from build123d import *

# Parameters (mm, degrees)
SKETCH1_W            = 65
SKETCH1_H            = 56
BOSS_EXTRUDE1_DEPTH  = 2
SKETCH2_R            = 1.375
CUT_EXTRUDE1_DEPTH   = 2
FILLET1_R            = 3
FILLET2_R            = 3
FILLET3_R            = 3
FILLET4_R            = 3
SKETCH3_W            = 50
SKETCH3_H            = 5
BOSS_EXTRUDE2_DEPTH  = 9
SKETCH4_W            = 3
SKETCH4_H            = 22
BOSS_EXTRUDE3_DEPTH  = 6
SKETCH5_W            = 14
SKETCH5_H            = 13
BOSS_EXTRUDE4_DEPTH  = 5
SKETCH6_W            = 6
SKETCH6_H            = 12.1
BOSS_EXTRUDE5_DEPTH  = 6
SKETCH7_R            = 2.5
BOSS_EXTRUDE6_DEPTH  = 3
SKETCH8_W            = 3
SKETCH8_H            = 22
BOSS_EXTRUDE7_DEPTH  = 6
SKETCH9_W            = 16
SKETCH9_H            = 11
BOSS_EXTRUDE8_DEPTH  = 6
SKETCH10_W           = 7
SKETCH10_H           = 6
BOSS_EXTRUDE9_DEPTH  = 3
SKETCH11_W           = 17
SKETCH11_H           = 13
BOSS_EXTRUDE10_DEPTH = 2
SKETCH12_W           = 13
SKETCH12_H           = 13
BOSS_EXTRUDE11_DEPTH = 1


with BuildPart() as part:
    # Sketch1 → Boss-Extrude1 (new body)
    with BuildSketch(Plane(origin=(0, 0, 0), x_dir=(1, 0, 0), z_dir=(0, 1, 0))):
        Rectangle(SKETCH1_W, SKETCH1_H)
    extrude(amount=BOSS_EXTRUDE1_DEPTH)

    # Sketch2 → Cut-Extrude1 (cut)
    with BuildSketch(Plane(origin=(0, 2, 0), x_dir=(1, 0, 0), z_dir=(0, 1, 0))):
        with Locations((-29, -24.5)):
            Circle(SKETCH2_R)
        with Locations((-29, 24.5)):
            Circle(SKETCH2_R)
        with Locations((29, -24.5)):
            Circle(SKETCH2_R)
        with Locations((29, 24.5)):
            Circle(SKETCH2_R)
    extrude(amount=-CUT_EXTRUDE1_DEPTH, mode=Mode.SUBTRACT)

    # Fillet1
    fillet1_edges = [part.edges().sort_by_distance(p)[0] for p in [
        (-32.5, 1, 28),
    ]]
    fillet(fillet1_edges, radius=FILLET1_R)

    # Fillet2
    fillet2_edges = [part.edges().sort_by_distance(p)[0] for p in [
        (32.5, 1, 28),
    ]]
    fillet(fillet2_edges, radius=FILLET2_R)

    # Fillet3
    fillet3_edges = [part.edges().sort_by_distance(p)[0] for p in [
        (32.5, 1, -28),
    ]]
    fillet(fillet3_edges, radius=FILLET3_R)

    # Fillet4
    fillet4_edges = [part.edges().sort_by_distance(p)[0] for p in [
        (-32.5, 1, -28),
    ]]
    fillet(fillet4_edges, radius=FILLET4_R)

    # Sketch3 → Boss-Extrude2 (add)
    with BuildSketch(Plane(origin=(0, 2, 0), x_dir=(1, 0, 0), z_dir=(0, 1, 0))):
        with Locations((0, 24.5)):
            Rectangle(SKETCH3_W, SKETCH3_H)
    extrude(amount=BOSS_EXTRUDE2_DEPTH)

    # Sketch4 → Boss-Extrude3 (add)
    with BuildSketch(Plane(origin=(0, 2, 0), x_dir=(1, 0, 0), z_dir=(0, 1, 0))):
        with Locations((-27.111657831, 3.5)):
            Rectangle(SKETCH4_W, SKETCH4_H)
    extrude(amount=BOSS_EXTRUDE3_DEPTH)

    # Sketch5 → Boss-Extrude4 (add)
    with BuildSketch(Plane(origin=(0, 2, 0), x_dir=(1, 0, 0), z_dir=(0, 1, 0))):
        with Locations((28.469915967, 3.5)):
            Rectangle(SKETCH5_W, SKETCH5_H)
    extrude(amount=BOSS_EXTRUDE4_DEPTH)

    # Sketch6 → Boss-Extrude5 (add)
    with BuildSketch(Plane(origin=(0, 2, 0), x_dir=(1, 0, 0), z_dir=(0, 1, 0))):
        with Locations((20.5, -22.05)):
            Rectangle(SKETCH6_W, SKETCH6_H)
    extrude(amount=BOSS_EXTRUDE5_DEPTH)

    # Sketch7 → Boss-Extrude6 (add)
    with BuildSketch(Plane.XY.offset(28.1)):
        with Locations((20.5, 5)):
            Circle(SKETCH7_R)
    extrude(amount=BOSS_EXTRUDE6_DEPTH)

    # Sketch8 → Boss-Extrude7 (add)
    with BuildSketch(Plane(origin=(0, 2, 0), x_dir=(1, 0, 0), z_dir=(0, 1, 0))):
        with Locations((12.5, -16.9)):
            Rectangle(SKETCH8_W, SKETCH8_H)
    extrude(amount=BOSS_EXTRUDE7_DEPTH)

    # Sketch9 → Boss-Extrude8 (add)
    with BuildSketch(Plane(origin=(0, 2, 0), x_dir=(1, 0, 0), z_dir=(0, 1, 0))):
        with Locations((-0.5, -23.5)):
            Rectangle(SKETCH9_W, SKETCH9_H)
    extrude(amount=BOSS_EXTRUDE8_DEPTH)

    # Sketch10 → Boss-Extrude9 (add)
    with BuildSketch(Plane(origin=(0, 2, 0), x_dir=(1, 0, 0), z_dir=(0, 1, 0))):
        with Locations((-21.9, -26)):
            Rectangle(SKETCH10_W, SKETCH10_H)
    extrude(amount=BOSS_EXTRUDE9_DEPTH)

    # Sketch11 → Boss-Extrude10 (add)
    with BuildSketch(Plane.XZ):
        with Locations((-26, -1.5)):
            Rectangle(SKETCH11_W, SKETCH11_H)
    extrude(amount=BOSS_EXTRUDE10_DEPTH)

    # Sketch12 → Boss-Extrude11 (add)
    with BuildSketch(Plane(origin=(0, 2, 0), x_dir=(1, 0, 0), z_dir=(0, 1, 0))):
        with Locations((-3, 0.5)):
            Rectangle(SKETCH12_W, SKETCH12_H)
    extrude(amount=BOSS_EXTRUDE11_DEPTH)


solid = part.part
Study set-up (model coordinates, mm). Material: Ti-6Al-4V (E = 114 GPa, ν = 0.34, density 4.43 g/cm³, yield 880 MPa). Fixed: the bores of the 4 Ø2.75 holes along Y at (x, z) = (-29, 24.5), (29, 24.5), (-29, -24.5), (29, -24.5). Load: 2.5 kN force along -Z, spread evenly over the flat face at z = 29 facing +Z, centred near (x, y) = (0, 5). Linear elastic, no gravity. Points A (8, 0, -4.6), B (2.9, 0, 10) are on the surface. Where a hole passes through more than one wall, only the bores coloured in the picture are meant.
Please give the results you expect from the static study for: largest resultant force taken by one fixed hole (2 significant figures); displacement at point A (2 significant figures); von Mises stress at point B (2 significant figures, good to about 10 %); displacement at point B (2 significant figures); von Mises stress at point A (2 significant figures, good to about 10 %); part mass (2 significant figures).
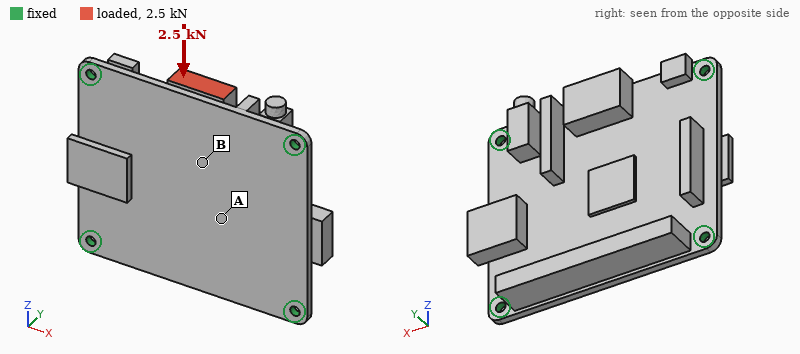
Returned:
810 N
0.070 mm
88 MPa
0.063 mm
36 MPa
60 g
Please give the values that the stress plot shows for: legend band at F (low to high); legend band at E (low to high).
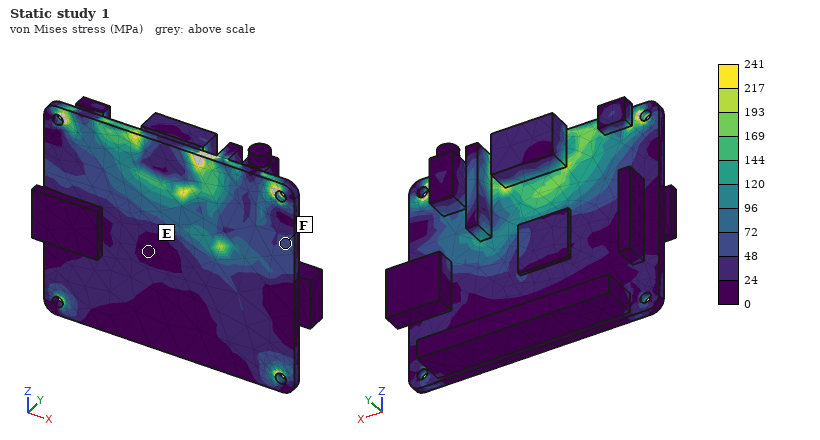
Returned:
48 to 72 MPa
0 to 24 MPa
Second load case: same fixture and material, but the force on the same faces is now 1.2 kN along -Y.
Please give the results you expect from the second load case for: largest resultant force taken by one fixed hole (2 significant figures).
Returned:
760 N
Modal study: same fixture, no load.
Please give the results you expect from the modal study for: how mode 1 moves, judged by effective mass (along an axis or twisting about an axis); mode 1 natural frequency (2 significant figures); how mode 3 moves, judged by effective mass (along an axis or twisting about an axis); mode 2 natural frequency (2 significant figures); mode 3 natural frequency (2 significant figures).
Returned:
along Y
2500 Hz
twisting about Z
3600 Hz
4500 Hz
